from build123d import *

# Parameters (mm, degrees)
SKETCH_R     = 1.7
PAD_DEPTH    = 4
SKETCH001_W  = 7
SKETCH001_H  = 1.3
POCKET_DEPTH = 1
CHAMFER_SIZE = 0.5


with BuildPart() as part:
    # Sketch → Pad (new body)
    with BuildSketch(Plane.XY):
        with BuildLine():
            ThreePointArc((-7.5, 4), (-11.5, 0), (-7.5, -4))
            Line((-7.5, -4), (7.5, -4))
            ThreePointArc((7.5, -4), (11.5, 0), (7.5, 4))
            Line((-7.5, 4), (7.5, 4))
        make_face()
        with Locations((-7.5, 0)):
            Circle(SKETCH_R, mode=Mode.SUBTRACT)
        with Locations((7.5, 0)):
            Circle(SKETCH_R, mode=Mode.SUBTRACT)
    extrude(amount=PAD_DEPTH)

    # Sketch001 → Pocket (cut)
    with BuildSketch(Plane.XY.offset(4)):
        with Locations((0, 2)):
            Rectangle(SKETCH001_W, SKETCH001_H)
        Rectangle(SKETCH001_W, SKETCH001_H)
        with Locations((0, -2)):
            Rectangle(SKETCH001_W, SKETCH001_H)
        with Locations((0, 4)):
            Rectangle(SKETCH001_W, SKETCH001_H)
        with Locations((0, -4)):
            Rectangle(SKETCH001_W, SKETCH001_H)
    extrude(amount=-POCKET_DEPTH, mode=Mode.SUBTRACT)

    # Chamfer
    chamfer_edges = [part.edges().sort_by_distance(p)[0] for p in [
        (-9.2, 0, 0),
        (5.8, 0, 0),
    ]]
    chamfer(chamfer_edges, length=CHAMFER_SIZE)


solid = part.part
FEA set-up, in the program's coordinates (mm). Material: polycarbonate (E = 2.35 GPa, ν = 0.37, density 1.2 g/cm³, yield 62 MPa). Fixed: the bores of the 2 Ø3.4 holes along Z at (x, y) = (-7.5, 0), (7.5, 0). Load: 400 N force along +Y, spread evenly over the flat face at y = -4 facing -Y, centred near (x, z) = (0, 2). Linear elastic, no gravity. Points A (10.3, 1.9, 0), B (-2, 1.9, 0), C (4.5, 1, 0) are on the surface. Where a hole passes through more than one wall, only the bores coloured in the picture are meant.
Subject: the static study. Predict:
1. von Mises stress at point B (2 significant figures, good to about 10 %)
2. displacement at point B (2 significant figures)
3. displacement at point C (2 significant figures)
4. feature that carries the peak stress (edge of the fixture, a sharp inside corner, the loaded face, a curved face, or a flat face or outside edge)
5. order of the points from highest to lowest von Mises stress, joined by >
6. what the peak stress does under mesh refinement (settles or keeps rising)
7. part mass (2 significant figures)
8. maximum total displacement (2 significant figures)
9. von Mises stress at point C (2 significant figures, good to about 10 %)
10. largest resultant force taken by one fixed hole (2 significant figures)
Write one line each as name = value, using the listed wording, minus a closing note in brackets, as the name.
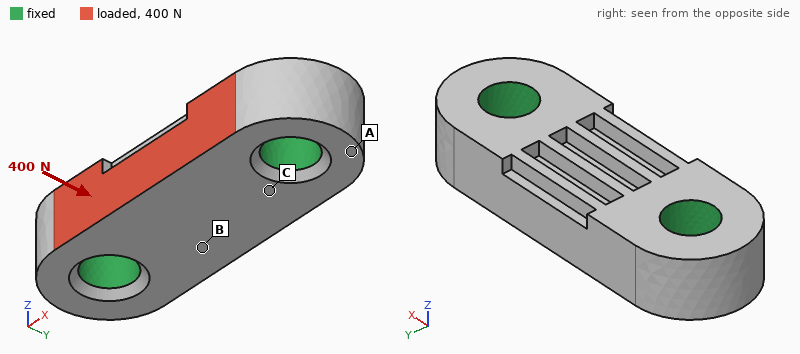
von Mises stress at point B = 5.1 MPa
displacement at point B = 33 µm
displacement at point C = 18 µm
feature that carries the peak stress = edge of the fixture
order of the points from highest to lowest von Mises stress, joined by > = C > B > A
what the peak stress does under mesh refinement = keeps rising
part mass = 0.68 g
maximum total displacement = 49 µm
von Mises stress at point C = 10 MPa
largest resultant force taken by one fixed hole = 200 N
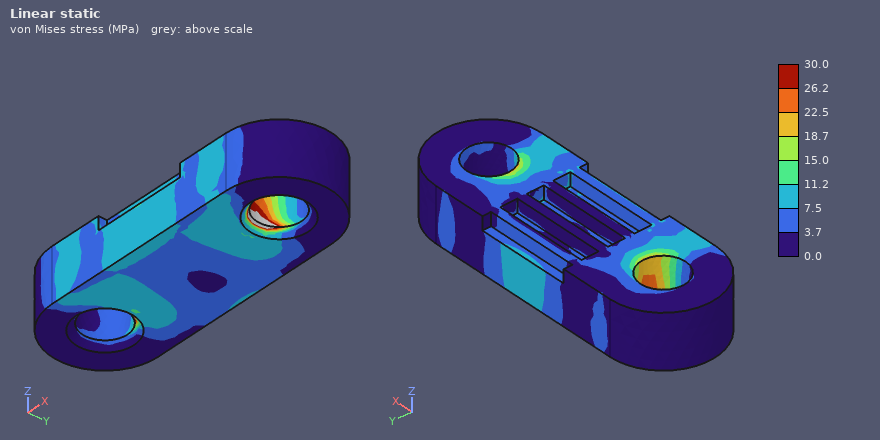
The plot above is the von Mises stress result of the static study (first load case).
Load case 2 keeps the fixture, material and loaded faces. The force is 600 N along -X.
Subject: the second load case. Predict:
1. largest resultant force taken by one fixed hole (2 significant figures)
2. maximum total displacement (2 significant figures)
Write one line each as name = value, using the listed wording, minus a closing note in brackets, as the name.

largest resultant force taken by one fixed hole = 320 N
maximum total displacement = 53 µm
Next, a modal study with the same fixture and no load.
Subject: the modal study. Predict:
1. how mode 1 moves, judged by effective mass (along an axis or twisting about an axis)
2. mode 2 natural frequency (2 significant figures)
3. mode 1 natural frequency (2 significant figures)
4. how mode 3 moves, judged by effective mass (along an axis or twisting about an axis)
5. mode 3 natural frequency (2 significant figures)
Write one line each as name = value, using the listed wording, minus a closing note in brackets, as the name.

how mode 1 moves, judged by effective mass = along Z
mode 2 natural frequency = 24 kHz
mode 1 natural frequency = 22 kHz
how mode 3 moves, judged by effective mass = along Y
mode 3 natural frequency = 26 kHz
